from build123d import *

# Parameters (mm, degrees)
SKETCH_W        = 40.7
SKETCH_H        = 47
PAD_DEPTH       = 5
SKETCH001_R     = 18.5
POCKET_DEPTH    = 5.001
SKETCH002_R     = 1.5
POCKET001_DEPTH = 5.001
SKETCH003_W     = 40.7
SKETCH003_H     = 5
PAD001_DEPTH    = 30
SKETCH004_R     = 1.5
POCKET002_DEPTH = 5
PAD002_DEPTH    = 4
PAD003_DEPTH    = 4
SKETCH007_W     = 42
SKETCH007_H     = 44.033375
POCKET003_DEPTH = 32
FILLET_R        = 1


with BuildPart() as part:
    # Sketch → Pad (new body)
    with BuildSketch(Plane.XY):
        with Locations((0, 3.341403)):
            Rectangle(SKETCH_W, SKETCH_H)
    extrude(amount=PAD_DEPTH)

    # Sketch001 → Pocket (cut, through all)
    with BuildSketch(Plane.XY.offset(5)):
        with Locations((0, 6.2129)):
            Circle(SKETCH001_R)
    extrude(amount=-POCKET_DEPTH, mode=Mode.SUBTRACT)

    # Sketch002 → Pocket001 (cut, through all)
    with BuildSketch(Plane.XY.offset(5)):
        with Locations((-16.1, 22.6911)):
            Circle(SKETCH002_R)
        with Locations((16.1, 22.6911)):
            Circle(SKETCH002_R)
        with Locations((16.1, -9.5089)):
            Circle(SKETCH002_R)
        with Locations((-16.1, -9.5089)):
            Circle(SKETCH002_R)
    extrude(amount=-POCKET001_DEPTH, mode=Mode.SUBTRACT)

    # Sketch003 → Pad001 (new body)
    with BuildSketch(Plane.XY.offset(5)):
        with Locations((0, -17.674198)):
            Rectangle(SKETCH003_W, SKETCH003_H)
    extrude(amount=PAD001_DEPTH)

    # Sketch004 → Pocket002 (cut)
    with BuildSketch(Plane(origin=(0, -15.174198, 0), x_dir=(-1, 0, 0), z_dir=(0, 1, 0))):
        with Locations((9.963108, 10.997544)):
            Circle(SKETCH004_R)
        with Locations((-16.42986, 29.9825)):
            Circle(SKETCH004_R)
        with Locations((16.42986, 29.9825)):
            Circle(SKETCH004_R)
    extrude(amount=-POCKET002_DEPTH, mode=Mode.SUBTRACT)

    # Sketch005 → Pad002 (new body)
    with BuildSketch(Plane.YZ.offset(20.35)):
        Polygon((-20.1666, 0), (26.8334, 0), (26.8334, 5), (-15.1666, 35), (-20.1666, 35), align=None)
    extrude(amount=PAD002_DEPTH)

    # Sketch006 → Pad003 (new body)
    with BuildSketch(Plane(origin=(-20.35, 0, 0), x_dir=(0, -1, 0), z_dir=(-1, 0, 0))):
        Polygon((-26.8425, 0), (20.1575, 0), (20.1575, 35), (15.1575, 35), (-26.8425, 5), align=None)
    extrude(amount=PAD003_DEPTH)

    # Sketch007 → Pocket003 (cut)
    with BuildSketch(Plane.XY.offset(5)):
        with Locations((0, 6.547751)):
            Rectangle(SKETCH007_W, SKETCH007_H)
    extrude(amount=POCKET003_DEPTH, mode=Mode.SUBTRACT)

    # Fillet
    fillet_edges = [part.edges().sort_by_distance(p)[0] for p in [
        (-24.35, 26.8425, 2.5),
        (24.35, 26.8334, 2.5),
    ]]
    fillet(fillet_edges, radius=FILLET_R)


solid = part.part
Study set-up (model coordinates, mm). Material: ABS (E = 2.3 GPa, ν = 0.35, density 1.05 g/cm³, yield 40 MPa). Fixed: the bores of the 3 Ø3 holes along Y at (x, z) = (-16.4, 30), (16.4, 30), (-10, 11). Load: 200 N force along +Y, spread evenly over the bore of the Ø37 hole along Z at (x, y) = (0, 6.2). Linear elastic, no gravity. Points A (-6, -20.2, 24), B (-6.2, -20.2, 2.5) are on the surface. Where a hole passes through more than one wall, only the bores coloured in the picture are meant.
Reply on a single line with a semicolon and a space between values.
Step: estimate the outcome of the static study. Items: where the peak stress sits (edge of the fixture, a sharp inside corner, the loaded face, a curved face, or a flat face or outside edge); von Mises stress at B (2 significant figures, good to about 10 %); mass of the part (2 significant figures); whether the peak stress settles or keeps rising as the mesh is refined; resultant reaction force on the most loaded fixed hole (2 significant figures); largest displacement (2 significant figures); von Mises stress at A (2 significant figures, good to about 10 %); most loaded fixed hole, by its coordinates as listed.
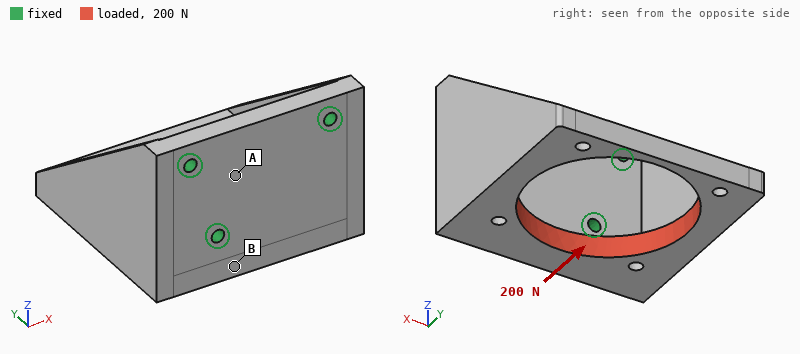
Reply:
edge of the fixture; 6.0 MPa; 18 g; keeps rising; 200 N; 0.91 mm; 2.5 MPa; (-10, 11)
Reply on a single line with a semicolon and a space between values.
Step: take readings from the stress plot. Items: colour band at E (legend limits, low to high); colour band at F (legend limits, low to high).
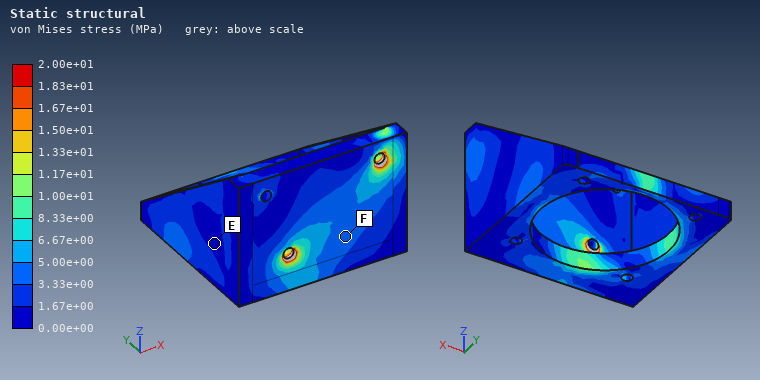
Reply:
0.00e+00 to 1.67e+00 MPa; 3.33e+00 to 5.00e+00 MPa
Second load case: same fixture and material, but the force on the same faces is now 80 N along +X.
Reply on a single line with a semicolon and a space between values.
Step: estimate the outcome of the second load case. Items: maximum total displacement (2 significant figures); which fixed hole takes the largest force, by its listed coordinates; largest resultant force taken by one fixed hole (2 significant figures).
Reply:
0.74 mm; (-10, 11); 75 N
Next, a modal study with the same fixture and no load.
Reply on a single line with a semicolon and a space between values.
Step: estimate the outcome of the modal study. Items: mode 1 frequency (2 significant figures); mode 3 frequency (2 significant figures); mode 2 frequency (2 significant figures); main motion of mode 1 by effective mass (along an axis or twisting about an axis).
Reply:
650 Hz; 1800 Hz; 1200 Hz; along X
